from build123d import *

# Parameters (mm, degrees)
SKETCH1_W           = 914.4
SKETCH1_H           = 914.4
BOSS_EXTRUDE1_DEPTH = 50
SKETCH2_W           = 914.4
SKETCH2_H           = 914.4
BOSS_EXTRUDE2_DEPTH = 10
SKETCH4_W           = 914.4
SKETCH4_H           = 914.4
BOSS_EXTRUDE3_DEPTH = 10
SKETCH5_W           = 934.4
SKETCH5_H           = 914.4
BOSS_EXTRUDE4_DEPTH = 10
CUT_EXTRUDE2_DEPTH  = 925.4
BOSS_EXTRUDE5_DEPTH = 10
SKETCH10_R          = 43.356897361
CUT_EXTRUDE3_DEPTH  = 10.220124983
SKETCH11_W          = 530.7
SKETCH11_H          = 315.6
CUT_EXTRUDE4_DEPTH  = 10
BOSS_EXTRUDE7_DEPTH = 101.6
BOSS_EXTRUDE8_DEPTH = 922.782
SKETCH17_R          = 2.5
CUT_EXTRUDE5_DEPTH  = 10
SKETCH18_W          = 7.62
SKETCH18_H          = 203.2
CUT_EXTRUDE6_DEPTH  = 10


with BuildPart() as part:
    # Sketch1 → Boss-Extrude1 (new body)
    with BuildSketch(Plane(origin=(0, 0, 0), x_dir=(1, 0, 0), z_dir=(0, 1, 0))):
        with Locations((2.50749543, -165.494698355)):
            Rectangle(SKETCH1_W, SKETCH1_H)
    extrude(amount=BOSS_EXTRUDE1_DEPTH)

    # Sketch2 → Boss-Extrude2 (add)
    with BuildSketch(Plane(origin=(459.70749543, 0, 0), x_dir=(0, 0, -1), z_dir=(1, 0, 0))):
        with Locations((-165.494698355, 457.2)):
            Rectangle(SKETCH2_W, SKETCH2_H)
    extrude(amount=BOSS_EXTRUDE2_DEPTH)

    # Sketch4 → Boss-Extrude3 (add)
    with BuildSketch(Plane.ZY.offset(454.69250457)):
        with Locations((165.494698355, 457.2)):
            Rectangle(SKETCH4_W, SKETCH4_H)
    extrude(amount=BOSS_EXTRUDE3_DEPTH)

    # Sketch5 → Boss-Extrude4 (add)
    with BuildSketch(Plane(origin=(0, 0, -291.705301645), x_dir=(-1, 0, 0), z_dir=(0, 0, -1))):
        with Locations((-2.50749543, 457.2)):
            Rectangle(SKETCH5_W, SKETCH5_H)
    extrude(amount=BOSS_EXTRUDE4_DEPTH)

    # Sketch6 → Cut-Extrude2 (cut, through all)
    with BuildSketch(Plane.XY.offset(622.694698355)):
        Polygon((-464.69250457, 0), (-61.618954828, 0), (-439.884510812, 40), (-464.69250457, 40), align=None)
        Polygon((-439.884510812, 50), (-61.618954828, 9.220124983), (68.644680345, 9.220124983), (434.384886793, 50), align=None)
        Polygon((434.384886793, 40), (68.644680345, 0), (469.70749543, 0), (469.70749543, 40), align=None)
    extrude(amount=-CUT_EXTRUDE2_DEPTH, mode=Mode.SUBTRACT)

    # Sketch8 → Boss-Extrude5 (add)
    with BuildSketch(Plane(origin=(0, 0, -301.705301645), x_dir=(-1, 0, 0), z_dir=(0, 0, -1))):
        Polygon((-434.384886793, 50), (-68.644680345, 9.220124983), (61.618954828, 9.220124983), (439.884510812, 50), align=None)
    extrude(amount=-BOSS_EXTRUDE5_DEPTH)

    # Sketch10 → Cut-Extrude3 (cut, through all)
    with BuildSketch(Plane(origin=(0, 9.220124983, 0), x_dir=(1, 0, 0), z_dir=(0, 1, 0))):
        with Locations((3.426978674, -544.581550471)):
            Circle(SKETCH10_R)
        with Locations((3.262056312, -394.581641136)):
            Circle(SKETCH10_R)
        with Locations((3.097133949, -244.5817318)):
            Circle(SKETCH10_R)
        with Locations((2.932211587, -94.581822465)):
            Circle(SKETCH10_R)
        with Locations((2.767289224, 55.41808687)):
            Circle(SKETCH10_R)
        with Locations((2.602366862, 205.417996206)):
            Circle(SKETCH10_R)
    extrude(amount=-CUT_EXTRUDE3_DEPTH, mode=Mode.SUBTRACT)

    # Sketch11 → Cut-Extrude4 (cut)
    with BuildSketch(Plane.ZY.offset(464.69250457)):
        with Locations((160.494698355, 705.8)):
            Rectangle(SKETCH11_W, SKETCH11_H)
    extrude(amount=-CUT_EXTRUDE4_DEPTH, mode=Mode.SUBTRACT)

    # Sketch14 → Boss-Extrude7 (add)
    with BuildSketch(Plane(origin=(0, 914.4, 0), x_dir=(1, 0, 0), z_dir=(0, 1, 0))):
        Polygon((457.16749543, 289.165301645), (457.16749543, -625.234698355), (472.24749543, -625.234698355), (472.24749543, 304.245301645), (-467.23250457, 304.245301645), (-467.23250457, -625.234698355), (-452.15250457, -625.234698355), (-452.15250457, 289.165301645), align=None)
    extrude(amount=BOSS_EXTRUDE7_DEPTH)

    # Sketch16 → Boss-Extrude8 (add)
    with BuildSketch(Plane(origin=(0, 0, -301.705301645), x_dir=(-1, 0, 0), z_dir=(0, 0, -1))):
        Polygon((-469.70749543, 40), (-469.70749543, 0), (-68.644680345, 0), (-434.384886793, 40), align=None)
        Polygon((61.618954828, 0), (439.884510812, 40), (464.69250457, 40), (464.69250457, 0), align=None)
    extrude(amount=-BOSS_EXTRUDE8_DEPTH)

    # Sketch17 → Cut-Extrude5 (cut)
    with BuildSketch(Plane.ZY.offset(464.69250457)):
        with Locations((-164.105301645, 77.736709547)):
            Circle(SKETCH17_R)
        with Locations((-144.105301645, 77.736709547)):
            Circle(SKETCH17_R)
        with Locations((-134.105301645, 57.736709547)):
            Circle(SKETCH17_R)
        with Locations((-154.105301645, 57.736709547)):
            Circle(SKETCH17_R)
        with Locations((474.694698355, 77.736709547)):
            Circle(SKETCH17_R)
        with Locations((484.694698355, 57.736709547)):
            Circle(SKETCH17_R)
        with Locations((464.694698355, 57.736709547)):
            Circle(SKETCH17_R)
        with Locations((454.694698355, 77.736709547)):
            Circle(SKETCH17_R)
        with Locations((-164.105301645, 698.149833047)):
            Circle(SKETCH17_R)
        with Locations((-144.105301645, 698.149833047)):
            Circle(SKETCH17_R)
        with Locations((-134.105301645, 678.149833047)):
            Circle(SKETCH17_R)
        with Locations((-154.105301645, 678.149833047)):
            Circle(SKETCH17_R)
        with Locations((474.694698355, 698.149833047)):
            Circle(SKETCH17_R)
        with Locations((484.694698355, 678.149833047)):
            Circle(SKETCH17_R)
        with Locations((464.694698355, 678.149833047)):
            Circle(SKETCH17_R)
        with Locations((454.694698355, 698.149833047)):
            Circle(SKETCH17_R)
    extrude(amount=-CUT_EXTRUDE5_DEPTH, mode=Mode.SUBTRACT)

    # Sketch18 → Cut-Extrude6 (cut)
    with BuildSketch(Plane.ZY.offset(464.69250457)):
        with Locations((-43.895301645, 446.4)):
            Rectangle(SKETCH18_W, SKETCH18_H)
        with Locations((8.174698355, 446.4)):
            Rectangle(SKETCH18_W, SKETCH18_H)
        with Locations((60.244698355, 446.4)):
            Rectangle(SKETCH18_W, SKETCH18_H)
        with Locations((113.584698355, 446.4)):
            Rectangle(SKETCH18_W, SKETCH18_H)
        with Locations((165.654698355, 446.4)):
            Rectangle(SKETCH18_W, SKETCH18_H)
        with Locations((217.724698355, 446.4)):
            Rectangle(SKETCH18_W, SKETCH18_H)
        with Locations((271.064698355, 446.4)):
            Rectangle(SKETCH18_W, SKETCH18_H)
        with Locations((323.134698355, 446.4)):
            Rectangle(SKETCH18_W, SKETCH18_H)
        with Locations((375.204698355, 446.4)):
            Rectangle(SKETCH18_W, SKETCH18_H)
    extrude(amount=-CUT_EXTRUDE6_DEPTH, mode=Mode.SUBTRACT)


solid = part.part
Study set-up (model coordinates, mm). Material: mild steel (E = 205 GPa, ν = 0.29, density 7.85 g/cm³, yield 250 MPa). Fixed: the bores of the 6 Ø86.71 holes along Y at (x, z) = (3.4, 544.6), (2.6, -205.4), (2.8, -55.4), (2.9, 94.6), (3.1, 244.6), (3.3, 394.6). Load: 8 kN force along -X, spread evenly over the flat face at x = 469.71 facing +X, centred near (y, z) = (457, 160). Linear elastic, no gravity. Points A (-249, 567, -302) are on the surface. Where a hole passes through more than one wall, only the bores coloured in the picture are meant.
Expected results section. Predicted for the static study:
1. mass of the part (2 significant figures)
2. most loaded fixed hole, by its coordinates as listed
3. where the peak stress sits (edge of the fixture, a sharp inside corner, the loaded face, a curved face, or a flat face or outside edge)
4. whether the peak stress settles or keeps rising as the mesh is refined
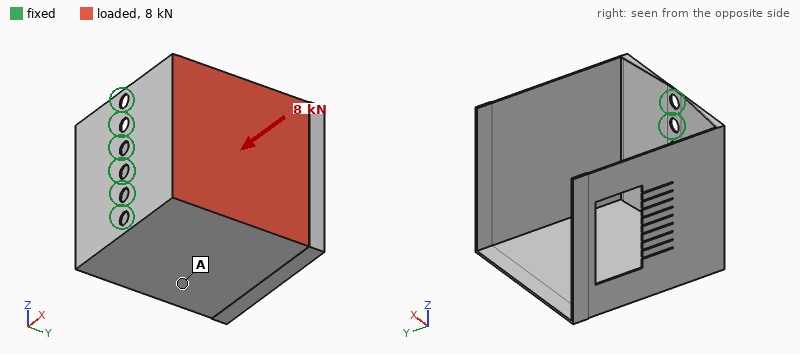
400 kg
(2.6, -205.4)
edge of the fixture
keeps rising
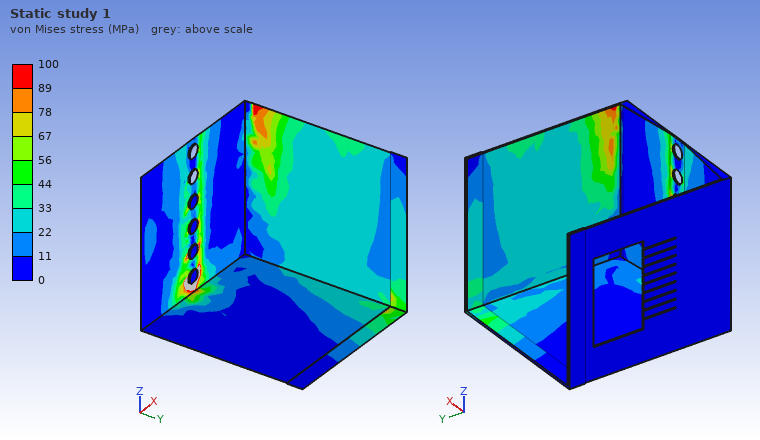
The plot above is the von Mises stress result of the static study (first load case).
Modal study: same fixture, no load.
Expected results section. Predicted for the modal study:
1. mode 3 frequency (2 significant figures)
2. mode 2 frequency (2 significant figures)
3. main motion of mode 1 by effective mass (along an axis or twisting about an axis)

24 Hz
16 Hz
along X
